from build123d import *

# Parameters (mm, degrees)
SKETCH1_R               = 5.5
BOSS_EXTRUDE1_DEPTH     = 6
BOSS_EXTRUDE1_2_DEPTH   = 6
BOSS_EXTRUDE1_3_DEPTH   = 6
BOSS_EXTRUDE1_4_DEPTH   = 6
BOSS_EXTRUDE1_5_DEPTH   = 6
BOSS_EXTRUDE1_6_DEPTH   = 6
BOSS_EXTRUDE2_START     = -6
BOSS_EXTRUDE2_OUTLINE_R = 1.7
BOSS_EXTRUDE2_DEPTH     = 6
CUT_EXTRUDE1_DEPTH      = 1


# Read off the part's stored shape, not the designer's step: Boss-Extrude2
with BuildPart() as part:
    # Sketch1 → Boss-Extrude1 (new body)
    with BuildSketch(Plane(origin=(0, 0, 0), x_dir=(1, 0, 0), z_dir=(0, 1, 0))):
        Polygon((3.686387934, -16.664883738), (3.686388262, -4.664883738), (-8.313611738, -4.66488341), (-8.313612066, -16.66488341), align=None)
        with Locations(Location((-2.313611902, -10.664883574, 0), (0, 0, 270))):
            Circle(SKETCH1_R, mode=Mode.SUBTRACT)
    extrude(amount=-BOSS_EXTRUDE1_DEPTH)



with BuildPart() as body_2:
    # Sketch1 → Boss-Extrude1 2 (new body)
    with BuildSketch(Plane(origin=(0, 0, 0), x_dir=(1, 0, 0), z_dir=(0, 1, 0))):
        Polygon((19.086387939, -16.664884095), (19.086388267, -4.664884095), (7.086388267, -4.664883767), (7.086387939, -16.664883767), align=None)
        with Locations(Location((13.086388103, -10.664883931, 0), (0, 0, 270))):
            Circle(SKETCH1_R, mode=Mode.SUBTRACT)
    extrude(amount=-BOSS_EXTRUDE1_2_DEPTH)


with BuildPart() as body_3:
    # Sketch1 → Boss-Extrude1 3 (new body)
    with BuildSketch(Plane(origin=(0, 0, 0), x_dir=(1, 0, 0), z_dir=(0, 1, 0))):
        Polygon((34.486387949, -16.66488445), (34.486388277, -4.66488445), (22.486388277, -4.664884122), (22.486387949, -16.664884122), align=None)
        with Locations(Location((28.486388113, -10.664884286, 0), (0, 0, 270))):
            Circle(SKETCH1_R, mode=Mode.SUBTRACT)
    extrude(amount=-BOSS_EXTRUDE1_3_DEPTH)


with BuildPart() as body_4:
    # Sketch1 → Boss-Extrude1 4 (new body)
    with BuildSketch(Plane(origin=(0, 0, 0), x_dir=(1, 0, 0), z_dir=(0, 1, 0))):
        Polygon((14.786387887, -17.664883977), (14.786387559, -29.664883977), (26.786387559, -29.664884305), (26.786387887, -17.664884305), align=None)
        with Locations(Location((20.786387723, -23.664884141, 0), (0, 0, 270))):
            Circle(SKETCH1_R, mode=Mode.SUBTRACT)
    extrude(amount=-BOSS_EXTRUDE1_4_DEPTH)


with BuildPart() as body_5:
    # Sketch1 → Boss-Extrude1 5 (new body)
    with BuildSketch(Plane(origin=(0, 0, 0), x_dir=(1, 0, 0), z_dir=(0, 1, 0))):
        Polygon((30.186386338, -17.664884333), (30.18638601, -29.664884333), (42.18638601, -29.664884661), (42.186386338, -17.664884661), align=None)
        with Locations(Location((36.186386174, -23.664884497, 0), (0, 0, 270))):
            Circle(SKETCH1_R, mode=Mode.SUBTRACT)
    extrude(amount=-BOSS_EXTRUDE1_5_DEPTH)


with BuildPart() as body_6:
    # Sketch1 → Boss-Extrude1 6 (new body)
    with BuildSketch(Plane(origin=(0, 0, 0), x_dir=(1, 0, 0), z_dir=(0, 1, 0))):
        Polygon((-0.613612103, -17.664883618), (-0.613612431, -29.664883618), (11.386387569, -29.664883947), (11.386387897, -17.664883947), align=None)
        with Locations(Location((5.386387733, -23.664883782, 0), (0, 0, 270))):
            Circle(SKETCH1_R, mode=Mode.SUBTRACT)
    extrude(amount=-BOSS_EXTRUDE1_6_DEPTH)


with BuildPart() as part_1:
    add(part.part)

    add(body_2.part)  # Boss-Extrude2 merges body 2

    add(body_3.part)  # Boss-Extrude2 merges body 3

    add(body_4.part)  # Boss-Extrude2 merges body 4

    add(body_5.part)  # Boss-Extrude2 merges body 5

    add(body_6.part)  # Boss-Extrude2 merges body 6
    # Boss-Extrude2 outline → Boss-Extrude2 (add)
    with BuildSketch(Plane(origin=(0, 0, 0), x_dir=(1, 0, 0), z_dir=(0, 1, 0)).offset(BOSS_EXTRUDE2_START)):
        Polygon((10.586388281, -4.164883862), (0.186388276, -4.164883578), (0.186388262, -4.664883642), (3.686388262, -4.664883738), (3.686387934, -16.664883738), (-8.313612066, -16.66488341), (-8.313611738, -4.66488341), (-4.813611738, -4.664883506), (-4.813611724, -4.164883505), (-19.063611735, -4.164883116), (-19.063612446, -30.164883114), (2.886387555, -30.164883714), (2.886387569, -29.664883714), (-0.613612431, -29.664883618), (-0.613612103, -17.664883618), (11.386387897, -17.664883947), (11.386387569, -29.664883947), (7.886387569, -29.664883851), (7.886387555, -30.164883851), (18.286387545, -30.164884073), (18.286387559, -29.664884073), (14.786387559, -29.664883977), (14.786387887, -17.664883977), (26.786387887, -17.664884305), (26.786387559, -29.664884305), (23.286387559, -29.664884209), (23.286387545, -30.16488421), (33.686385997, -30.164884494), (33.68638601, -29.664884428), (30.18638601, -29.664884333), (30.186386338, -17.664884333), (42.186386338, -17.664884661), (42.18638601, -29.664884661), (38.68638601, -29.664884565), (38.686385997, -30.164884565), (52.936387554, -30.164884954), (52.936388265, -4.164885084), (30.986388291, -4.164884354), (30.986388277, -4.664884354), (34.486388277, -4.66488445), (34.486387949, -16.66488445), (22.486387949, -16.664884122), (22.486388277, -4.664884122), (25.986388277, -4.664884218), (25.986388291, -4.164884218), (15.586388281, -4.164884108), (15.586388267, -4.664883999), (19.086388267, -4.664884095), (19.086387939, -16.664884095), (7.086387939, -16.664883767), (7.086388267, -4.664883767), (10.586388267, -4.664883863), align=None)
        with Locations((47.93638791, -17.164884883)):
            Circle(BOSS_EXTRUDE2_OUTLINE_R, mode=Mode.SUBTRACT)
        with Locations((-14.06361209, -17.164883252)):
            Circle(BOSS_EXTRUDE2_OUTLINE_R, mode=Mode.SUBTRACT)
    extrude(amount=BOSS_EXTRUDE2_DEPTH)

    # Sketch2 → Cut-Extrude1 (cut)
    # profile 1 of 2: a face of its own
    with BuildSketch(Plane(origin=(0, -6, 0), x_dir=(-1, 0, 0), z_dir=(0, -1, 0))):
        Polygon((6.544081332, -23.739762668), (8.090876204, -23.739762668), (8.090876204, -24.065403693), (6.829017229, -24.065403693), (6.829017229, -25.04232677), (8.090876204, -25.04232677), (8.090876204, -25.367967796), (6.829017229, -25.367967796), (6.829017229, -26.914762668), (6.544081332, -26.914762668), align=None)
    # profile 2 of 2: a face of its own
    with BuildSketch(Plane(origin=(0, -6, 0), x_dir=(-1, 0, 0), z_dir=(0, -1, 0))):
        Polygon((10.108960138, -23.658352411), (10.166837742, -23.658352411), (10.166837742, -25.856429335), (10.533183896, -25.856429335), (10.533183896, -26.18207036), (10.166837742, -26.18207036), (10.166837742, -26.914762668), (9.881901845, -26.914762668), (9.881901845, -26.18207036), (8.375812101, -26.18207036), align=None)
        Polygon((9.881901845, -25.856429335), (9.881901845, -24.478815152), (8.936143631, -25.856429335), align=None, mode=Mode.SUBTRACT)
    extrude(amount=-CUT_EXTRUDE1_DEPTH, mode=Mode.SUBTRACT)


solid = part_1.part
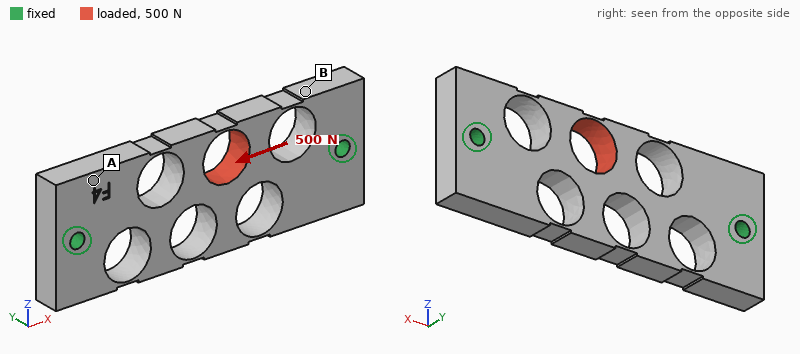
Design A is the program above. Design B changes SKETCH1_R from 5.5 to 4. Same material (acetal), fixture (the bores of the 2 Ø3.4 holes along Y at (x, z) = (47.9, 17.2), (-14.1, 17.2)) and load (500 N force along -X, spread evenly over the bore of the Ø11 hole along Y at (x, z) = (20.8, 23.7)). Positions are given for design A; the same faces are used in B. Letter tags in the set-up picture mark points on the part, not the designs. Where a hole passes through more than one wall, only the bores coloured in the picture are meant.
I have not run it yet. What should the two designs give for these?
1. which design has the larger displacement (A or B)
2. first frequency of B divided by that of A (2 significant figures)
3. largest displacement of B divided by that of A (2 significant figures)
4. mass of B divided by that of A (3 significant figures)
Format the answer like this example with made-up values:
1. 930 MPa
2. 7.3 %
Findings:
1. A
2. 1.00
3. 0.47
4. 1.21
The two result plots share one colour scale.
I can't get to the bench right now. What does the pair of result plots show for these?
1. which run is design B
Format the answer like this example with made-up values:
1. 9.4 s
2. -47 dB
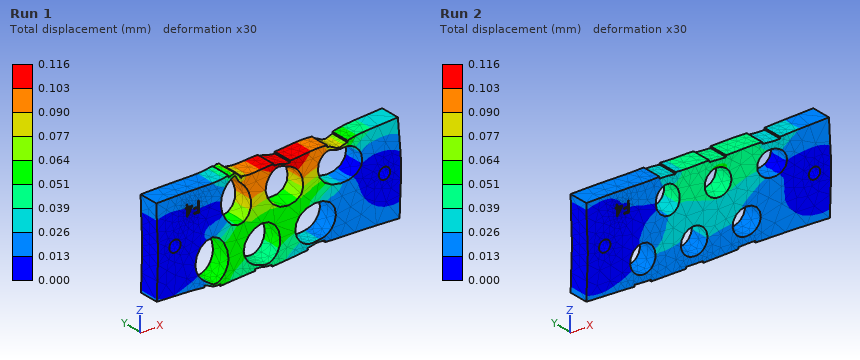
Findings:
1. Run 2
